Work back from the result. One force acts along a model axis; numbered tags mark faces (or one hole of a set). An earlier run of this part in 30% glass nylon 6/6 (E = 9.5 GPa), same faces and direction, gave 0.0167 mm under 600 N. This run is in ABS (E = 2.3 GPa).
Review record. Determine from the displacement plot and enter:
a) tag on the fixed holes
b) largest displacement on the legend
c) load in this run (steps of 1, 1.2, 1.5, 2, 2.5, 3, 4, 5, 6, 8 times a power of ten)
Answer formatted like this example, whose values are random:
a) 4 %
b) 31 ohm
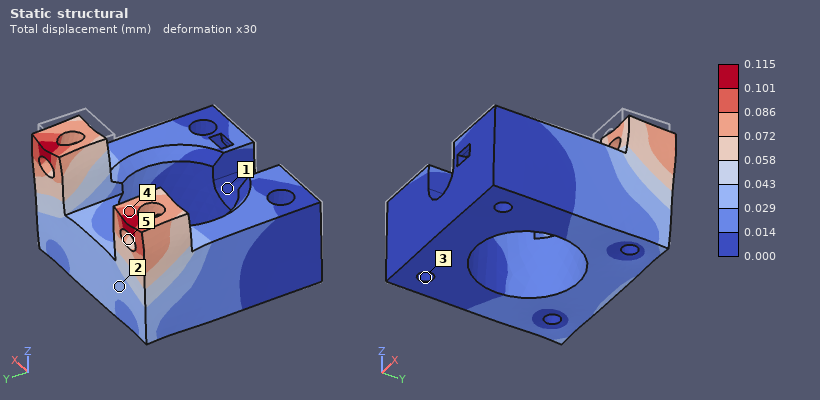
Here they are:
a) 3
b) 0.115 mm
c) 1 kN
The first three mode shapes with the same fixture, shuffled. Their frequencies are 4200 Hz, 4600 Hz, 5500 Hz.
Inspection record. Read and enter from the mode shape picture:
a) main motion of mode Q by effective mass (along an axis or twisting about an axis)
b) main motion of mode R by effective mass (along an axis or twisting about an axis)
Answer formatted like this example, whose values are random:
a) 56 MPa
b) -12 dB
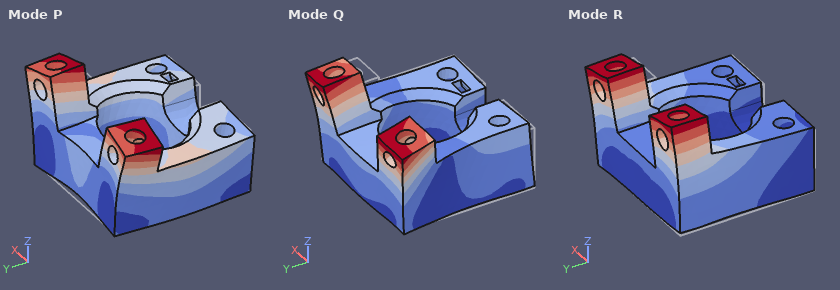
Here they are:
a) along Y
b) along X
